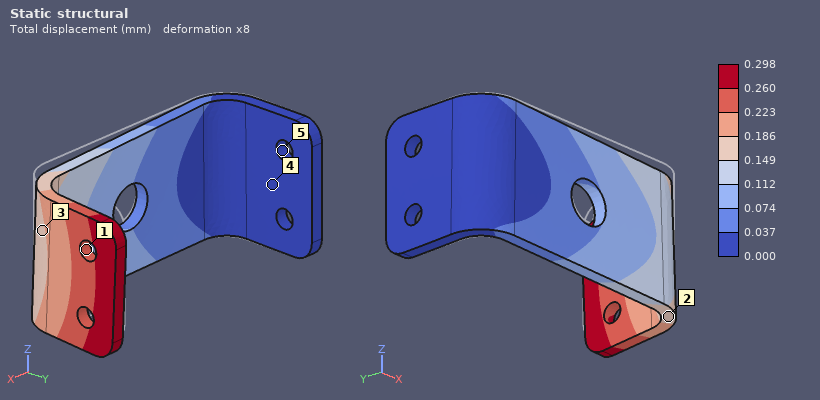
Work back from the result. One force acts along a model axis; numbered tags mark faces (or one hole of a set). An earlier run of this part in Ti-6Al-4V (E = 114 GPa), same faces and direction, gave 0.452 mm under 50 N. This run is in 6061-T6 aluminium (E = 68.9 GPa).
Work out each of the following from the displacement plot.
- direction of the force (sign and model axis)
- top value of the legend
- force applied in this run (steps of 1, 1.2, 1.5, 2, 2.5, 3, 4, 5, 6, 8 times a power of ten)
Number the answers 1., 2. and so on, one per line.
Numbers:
1. -Z
2. 0.298 mm
3. 20 N
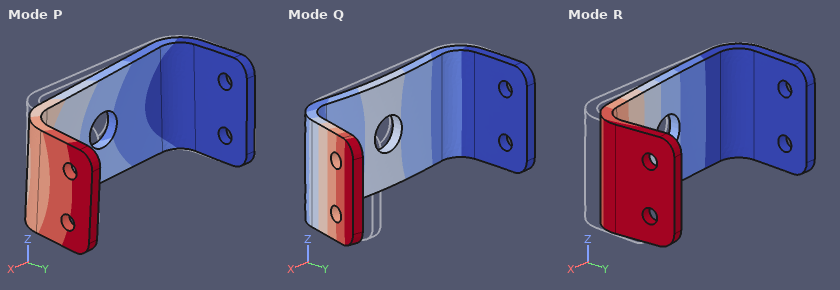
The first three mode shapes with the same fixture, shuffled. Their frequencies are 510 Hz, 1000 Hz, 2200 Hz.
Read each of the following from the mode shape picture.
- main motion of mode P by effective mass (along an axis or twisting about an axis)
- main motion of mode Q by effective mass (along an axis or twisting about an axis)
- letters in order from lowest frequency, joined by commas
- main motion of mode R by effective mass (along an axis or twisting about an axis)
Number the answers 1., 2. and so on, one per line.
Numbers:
1. along Z
2. along X
3. R, P, Q
4. along Y
